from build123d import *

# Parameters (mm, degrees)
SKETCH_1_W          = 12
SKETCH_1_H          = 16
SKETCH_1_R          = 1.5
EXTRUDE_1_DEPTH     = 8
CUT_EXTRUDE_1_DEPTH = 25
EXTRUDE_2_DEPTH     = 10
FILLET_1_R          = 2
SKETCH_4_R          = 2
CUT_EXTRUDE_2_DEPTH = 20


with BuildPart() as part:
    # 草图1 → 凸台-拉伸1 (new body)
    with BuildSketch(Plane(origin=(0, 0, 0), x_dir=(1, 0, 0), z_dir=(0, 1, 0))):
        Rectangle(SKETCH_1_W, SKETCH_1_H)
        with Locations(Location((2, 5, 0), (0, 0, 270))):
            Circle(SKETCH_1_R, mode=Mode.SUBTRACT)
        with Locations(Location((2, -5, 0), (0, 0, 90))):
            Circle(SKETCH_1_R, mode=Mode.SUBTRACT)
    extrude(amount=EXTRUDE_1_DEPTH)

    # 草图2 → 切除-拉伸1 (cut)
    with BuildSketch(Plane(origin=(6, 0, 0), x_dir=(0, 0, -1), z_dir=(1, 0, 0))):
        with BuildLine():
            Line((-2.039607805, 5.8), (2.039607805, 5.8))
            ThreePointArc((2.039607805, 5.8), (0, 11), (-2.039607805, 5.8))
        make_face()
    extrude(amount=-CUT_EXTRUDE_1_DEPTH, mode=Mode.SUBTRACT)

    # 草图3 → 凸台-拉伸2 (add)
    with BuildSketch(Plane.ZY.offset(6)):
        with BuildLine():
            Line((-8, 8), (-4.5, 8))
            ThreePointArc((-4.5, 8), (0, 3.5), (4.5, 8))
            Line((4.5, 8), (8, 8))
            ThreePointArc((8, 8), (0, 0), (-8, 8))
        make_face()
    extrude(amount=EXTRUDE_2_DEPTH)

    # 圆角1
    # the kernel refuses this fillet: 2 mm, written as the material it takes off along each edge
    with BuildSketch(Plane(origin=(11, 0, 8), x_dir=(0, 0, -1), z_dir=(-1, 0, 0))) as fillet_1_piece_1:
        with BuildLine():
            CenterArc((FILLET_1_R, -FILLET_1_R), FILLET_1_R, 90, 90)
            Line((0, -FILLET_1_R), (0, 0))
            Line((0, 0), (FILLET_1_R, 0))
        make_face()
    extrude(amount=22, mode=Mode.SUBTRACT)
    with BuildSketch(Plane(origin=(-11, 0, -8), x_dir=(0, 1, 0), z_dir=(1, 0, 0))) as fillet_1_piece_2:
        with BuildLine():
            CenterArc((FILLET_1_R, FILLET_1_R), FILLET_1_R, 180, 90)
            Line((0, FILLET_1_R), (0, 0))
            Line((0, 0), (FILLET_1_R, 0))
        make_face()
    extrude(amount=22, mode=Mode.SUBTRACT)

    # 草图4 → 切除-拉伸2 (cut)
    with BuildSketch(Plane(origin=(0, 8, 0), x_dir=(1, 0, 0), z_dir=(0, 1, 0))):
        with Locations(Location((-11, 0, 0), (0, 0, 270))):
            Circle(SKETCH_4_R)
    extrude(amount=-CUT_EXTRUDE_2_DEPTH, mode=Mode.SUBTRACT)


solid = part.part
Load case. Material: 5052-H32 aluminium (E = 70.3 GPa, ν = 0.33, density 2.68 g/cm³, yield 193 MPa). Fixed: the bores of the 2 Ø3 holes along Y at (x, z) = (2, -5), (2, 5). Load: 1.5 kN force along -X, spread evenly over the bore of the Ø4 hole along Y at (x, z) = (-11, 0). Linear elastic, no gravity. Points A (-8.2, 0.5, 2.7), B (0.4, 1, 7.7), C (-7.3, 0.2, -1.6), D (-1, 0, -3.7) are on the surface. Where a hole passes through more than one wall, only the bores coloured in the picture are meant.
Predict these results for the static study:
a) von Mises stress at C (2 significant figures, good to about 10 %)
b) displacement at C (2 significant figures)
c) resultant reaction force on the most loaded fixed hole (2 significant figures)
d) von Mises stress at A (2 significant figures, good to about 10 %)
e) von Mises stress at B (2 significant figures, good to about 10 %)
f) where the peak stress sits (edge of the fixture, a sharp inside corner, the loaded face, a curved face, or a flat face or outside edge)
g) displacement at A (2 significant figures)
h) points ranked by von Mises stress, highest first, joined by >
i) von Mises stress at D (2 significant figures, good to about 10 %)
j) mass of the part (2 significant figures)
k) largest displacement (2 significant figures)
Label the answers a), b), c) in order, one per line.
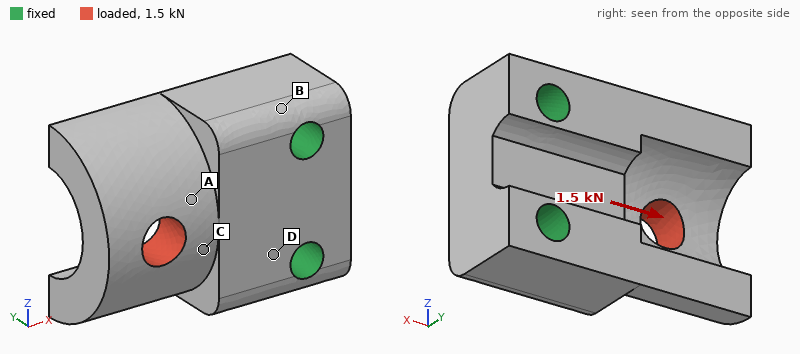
a) 55 MPa
b) 6.7 µm
c) 780 N
d) 67 MPa
e) 18 MPa
f) the loaded face
g) 7.6 µm
h) A > C > D > B
i) 41 MPa
j) 5.1 g
k) 20 µm
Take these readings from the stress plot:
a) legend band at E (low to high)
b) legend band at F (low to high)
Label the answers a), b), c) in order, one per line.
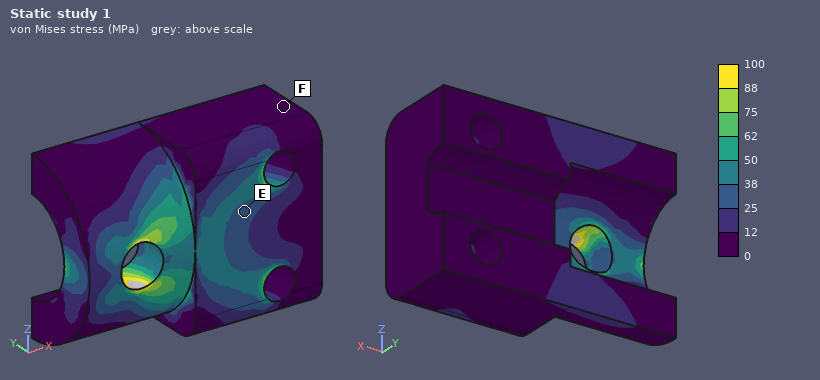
a) 25 to 38 MPa
b) 0 to 12 MPa
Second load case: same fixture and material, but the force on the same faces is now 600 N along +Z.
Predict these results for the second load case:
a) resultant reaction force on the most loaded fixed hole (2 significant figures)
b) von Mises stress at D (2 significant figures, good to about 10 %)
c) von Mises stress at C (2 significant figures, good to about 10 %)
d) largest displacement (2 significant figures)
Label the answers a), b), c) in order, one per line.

a) 700 N
b) 18 MPa
c) 21 MPa
d) 12 µm
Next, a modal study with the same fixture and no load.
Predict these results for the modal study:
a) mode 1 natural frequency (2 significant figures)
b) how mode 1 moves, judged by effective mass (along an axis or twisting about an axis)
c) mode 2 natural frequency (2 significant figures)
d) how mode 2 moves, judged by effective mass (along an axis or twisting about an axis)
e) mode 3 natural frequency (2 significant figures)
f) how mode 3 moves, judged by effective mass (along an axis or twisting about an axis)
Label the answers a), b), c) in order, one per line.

a) 22 kHz
b) along Y
c) 25 kHz
d) along Z
e) 37 kHz
f) along Z
